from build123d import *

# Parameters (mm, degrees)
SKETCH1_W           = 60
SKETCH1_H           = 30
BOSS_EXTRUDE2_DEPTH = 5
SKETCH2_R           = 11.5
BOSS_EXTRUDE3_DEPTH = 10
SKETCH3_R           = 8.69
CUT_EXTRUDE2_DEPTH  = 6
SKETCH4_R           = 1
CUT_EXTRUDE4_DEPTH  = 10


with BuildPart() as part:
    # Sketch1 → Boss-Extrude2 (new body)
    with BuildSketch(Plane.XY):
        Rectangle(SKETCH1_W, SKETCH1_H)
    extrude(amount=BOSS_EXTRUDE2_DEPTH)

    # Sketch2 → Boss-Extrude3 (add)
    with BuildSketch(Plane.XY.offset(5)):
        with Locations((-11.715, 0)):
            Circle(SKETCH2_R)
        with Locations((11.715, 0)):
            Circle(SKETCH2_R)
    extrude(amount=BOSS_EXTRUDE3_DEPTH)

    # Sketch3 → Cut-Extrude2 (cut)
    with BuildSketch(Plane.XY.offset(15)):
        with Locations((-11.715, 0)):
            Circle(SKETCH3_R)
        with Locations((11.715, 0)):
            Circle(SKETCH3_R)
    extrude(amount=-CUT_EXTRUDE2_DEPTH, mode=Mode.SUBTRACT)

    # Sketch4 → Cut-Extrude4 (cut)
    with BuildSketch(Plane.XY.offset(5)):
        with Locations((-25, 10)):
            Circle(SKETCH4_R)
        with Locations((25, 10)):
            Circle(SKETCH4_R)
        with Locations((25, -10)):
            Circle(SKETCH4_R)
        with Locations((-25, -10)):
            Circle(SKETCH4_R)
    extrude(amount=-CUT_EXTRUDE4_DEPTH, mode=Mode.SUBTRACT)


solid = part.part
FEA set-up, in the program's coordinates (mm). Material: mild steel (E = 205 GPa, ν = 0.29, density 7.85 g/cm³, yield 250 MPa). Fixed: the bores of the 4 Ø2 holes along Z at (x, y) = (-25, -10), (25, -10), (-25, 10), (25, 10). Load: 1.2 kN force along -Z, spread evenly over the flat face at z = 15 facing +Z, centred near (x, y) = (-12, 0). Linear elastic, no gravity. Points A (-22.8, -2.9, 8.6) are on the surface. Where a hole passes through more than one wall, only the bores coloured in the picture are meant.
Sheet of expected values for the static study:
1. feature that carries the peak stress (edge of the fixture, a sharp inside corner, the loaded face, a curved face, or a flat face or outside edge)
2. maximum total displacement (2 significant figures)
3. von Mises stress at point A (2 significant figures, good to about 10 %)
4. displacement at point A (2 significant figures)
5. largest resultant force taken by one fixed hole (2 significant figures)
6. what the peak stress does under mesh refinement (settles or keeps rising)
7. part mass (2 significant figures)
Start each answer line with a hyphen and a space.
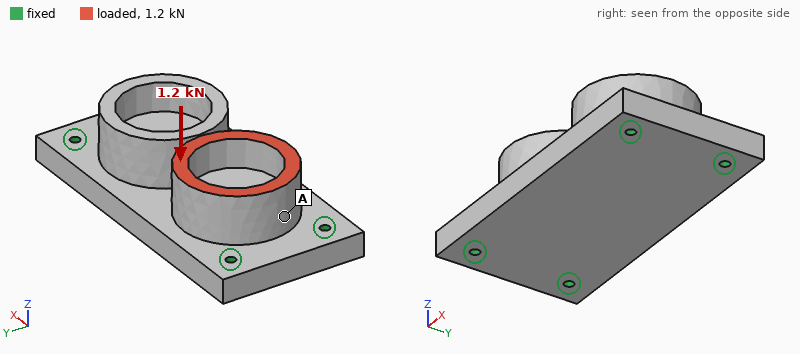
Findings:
- edge of the fixture
- 8.5 µm
- 5.7 MPa
- 2.4 µm
- 470 N
- keeps rising
- 110 g
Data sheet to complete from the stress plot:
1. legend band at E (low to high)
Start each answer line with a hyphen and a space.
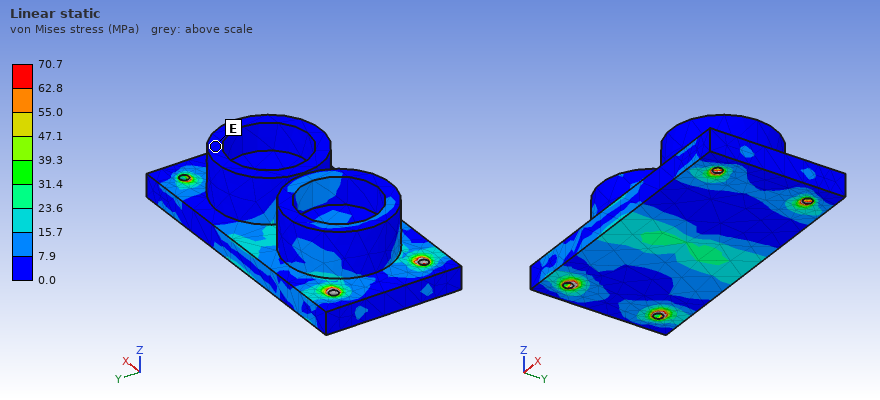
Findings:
- 0.0 to 7.9 MPa
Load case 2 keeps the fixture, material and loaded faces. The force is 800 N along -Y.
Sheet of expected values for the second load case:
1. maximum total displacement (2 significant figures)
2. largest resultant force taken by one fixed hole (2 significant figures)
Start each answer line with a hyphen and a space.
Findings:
- 5.6 µm
- 510 N
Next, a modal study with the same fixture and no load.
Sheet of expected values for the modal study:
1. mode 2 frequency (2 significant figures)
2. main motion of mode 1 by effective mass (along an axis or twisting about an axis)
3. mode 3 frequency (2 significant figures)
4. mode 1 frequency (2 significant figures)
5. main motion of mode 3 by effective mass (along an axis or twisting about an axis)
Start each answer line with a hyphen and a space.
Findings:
- 15 kHz
- along Z
- 20 kHz
- 7400 Hz
- along Y
